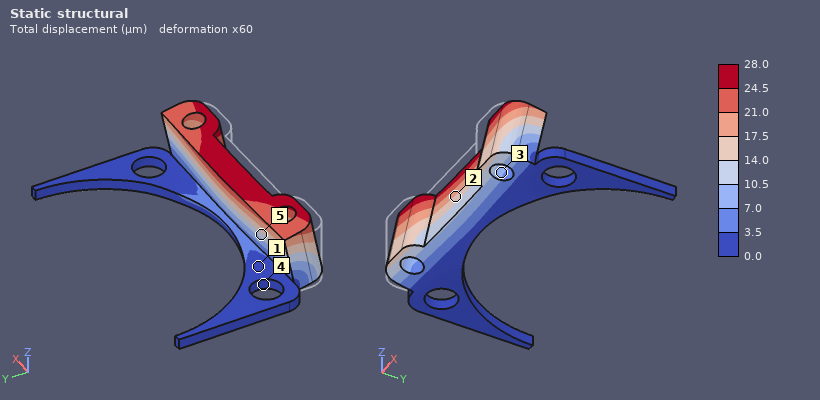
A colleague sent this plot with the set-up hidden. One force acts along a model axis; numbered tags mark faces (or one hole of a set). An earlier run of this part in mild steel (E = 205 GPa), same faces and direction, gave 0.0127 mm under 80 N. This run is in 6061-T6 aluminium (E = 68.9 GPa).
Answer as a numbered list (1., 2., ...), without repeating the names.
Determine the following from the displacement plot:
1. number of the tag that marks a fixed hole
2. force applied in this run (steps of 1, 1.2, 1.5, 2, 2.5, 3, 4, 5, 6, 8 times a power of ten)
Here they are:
1. 4
2. 60 N
